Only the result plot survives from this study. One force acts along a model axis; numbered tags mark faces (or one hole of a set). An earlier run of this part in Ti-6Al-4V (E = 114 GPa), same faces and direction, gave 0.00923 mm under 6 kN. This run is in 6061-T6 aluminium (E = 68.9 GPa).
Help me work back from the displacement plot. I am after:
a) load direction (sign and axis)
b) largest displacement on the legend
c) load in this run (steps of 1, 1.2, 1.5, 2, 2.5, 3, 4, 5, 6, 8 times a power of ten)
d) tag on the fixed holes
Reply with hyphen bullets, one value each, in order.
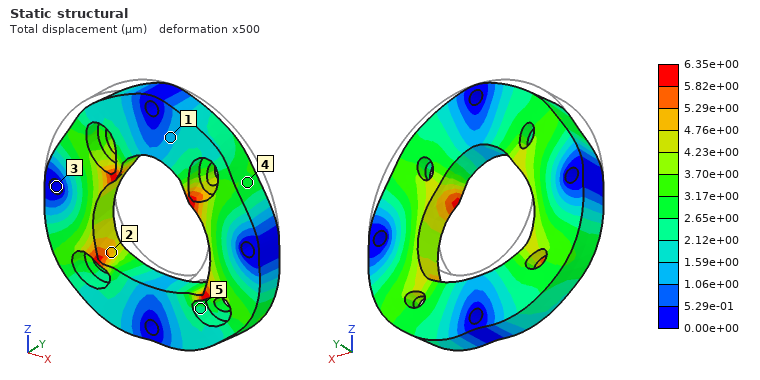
- -Z
- 6.35e+00 µm
- 2.5 kN
- 3
